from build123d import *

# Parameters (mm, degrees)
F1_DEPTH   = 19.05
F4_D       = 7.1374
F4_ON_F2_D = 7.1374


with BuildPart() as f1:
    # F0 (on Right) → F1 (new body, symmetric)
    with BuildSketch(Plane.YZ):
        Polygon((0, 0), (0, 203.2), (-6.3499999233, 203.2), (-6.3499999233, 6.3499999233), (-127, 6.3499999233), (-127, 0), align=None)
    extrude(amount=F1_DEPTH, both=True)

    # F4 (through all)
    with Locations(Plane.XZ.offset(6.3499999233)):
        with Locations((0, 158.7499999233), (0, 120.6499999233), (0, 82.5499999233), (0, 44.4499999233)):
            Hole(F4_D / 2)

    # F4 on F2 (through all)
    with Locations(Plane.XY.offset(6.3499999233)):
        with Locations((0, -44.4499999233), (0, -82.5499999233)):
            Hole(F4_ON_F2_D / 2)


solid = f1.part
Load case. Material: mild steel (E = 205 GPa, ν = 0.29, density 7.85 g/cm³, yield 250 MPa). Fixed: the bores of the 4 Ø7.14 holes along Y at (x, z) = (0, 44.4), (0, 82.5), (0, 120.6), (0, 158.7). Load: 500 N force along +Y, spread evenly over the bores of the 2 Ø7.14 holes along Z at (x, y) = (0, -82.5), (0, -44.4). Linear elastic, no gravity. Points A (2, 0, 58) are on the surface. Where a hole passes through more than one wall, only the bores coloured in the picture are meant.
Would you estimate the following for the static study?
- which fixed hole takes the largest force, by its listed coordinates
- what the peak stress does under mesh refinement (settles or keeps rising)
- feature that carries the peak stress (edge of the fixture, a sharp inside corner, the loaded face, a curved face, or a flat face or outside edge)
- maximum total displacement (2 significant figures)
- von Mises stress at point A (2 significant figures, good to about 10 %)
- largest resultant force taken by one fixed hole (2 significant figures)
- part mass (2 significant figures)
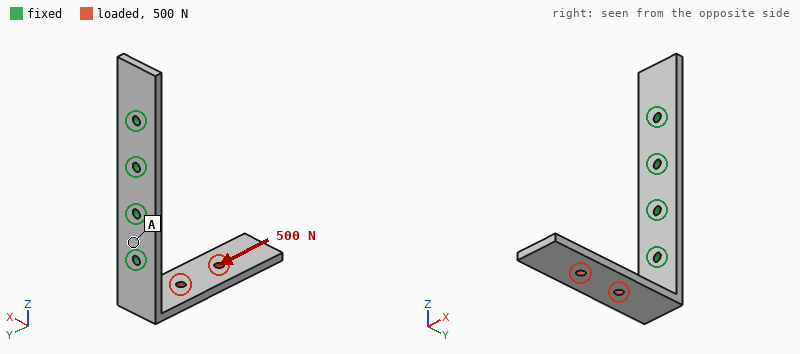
(0, 44.4)
keeps rising
edge of the fixture
0.32 mm
8.9 MPa
630 N
600 g
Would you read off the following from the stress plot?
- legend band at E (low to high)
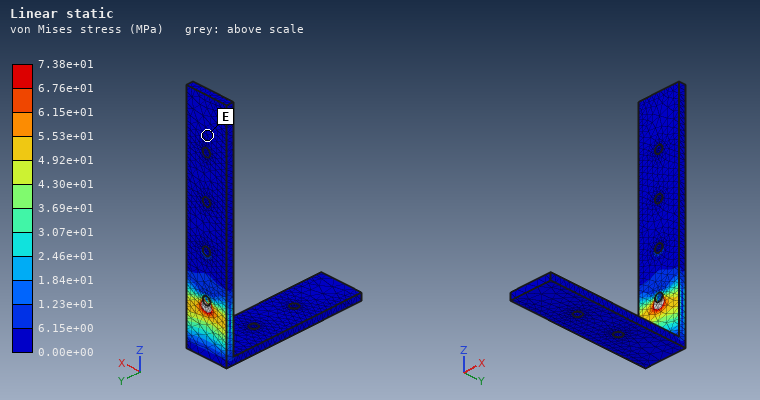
0.00e+00 to 6.15e+00 MPa
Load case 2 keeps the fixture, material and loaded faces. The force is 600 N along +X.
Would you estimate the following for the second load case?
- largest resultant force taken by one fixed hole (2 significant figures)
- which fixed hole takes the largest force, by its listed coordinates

1.0 kN
(0, 44.4)
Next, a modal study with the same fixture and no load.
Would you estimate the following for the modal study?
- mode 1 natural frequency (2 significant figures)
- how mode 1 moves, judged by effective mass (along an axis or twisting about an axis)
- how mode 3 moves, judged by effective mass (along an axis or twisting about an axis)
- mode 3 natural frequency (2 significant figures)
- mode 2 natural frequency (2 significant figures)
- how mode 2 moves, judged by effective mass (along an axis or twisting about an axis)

230 Hz
along Z
along Y
1100 Hz
360 Hz
along X
